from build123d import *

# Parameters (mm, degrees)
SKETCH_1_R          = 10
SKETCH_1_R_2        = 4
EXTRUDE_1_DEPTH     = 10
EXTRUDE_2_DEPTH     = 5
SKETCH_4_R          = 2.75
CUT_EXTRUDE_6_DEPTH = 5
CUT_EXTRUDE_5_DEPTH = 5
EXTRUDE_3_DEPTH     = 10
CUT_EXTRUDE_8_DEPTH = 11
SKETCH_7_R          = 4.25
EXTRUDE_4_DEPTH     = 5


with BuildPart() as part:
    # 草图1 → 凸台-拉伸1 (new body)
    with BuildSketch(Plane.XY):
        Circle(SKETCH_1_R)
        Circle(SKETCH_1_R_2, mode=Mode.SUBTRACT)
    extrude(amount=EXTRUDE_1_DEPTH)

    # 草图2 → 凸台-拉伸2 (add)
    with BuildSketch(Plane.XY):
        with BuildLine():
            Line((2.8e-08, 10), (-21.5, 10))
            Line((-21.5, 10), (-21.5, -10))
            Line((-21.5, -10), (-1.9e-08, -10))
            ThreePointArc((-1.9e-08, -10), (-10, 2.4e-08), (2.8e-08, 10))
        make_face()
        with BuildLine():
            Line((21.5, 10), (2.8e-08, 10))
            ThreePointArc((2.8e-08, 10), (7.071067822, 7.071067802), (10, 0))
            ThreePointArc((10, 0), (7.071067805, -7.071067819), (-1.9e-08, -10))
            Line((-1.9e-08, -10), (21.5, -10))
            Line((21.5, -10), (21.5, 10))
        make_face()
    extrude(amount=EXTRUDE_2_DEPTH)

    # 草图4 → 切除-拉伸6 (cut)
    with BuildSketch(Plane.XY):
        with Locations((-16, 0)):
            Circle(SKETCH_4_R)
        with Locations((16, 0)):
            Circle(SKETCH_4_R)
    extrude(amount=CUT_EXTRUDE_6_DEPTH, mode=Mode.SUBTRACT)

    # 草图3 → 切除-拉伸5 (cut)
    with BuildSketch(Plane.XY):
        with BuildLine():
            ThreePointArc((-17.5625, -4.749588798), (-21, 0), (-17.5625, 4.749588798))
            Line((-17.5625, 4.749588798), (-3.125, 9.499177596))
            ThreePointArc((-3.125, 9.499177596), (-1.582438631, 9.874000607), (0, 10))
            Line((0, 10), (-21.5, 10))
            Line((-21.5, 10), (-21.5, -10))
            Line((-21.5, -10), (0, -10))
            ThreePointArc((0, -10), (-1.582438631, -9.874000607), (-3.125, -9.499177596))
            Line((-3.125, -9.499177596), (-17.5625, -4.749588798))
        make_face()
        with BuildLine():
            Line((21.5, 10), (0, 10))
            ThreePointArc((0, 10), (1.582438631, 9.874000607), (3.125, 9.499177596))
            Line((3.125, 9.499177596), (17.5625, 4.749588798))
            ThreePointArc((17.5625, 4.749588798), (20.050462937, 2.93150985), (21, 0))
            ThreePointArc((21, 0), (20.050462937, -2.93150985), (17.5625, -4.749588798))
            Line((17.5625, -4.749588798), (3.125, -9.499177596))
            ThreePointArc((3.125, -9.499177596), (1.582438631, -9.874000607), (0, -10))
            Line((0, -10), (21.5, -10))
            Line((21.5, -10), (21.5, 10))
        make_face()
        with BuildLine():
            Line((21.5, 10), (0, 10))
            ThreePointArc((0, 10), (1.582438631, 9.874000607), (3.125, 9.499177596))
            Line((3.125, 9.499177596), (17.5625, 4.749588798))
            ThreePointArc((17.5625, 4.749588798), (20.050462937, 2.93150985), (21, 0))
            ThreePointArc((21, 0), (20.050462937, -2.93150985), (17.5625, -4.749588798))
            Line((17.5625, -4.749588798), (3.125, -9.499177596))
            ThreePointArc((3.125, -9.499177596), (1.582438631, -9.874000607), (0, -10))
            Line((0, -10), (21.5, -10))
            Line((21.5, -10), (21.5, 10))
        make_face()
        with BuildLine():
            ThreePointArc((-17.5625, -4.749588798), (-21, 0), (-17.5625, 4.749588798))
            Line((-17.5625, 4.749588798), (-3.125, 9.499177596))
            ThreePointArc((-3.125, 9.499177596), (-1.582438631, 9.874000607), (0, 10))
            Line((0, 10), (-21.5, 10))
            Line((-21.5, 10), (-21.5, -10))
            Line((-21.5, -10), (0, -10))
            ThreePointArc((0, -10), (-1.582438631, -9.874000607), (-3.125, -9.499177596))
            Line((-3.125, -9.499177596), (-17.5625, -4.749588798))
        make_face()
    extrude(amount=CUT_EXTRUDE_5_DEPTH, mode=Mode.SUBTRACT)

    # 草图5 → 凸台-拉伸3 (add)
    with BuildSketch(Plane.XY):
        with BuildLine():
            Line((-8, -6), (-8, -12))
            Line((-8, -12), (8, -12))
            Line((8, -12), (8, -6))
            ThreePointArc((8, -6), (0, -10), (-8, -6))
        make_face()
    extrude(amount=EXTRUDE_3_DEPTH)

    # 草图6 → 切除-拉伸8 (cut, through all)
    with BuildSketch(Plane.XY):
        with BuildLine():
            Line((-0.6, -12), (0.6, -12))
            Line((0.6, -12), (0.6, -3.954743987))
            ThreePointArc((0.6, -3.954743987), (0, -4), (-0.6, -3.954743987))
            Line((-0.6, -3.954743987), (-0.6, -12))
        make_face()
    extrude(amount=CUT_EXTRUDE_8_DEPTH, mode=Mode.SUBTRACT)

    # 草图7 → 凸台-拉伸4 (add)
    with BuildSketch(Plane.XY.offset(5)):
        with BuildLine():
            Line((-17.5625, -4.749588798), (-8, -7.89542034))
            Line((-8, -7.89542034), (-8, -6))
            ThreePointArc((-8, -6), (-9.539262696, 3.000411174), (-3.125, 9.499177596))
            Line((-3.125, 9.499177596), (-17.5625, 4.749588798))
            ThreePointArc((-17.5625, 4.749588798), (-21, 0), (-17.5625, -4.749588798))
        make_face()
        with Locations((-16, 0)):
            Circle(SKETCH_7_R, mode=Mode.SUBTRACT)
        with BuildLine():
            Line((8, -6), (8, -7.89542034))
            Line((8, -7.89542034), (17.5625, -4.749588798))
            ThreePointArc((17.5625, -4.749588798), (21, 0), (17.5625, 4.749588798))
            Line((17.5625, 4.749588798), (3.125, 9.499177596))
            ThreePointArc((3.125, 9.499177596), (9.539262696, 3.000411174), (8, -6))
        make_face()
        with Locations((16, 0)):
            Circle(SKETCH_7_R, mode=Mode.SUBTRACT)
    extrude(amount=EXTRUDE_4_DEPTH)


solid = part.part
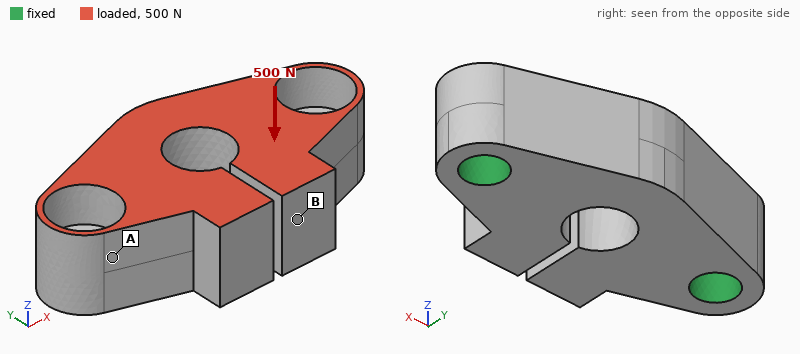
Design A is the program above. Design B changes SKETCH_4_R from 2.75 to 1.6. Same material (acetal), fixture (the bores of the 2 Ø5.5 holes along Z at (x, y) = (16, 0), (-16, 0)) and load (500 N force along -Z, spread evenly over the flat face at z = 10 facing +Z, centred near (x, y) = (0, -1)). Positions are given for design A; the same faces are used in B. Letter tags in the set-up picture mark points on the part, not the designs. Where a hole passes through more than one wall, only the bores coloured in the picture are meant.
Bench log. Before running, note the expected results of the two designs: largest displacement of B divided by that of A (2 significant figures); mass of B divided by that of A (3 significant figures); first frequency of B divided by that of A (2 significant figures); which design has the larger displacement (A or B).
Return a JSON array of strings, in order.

["1.4", "1.03", "0.82", "B"]
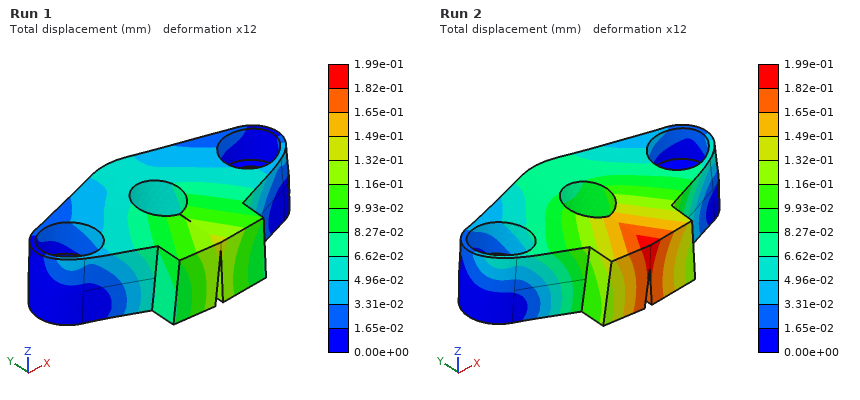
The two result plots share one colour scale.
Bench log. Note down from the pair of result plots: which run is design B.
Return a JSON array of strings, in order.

["Run 2"]
